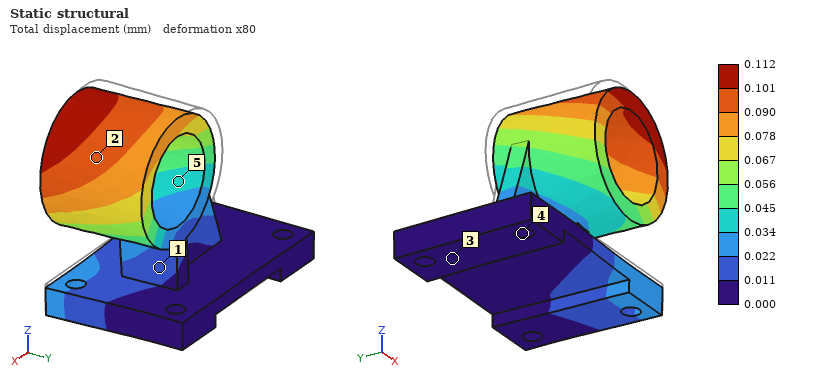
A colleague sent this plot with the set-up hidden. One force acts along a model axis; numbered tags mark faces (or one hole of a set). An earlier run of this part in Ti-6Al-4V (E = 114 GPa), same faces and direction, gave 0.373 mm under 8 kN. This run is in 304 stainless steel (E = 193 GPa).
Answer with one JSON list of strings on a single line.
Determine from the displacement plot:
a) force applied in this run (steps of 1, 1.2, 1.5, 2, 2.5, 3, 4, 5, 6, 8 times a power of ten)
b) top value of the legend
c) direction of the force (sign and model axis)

["4 kN", "0.112 mm", "+X"]
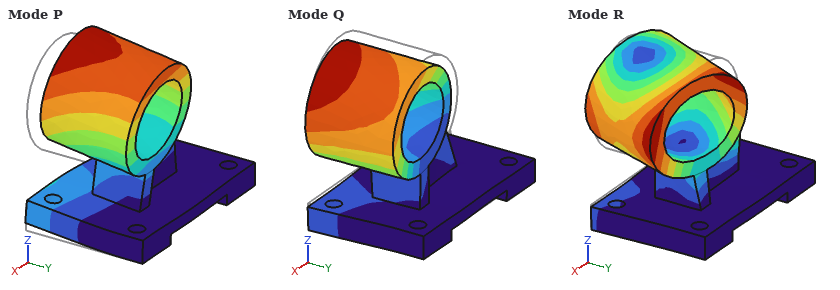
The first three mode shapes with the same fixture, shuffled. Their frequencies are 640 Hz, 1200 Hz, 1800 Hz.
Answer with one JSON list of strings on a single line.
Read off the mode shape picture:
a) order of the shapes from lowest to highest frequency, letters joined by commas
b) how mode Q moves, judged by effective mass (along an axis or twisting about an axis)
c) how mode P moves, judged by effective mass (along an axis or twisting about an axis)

["P, Q, R", "along X", "along Y"]
